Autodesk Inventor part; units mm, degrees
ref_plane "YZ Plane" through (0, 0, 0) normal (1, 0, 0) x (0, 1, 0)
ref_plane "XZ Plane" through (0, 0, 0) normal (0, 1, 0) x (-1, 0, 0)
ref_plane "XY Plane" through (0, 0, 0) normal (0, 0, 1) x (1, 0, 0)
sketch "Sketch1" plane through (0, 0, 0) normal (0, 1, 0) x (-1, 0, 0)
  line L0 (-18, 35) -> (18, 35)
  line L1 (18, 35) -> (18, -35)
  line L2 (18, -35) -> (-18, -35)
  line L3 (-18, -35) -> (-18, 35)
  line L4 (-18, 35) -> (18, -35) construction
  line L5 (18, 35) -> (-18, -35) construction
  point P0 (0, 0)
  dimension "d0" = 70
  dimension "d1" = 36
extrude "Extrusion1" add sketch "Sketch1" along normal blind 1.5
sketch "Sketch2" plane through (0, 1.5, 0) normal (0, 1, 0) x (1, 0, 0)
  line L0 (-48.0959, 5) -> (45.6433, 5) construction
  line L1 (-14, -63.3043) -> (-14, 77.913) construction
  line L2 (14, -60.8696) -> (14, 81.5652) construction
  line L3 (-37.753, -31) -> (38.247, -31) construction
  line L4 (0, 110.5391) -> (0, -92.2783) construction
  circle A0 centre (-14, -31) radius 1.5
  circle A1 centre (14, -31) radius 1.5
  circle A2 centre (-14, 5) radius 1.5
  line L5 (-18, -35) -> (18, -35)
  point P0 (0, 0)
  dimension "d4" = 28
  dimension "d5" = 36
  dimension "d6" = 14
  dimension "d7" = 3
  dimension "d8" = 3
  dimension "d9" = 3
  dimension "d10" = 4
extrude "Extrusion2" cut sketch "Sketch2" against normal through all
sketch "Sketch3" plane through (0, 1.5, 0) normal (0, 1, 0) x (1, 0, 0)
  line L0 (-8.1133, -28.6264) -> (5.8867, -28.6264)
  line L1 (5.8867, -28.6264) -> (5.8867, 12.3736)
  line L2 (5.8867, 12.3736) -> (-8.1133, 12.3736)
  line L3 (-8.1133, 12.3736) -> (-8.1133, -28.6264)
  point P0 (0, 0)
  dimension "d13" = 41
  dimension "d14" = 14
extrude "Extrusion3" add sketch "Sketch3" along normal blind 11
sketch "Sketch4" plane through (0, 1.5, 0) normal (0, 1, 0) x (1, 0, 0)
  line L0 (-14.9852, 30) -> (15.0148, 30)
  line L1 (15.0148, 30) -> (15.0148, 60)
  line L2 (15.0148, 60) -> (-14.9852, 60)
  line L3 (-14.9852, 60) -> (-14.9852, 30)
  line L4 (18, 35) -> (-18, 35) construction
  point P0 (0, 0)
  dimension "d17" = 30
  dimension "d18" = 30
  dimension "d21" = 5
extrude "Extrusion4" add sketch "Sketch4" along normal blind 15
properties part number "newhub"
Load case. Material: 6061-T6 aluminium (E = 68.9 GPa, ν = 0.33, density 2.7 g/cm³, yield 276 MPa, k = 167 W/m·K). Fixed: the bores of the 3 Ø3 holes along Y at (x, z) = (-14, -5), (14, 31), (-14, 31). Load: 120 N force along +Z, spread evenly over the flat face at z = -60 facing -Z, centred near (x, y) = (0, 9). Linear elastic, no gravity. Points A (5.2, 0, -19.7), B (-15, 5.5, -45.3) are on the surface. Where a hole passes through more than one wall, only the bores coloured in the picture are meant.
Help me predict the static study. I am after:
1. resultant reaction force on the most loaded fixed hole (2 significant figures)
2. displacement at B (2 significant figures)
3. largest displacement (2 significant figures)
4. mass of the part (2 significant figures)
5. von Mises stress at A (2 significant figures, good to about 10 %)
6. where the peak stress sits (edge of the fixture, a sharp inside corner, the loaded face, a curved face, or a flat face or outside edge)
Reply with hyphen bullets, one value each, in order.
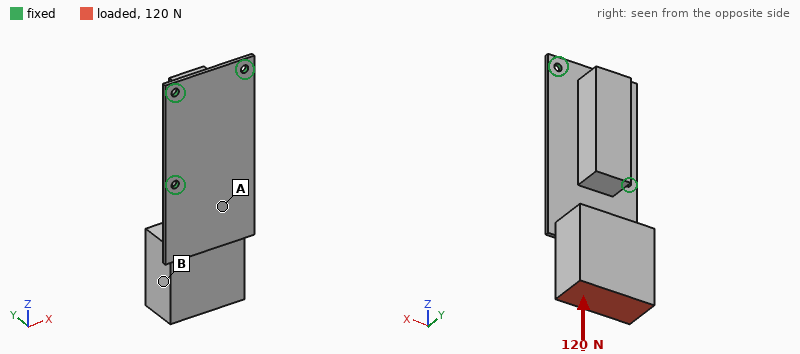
- 58 N
- 0.67 mm
- 1.1 mm
- 64 g
- 63 MPa
- a flat face or outside edge
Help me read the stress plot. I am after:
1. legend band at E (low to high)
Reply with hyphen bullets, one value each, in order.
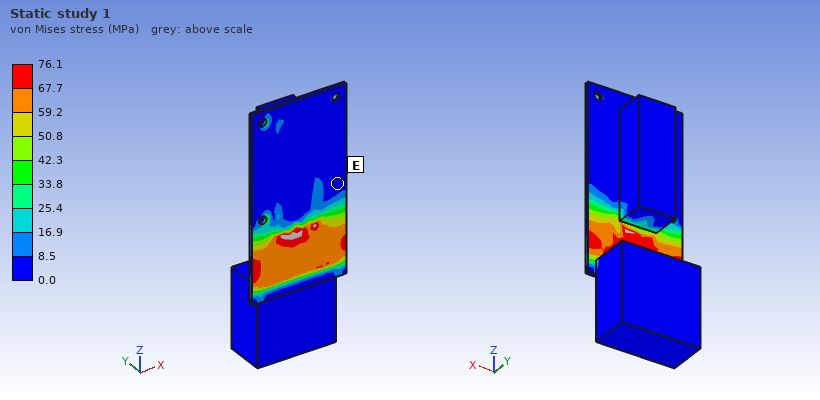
- 0.0 to 8.5 MPa
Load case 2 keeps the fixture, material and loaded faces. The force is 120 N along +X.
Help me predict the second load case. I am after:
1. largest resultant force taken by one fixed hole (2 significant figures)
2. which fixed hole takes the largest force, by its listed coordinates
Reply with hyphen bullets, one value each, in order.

- 260 N
- (-14, -5)
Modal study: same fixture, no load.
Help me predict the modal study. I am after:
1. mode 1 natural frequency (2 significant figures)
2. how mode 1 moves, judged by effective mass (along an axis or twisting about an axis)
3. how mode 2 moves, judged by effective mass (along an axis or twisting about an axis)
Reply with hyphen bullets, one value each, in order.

- 180 Hz
- along Y
- along X
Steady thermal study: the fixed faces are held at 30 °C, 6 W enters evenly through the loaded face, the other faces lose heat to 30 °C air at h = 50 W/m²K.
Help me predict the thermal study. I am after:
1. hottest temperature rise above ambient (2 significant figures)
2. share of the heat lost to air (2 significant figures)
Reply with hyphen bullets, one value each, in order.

- 14 K
- 51 %
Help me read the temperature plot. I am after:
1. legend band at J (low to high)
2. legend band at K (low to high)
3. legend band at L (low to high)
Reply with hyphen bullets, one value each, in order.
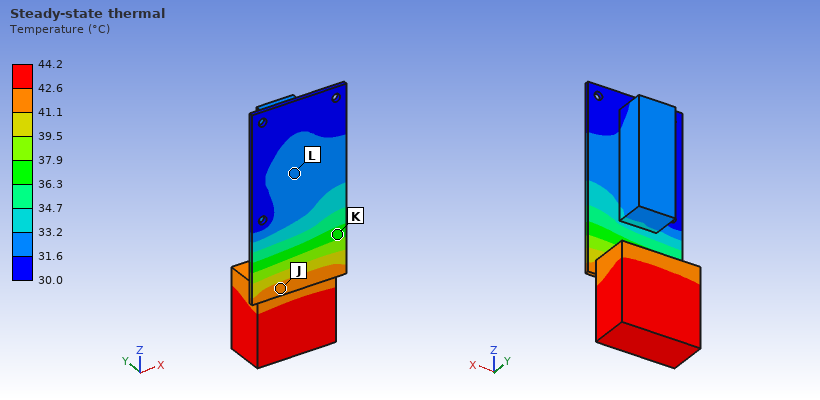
- 41.1 to 42.6 °C
- 36.3 to 37.9 °C
- 31.6 to 33.2 °C
